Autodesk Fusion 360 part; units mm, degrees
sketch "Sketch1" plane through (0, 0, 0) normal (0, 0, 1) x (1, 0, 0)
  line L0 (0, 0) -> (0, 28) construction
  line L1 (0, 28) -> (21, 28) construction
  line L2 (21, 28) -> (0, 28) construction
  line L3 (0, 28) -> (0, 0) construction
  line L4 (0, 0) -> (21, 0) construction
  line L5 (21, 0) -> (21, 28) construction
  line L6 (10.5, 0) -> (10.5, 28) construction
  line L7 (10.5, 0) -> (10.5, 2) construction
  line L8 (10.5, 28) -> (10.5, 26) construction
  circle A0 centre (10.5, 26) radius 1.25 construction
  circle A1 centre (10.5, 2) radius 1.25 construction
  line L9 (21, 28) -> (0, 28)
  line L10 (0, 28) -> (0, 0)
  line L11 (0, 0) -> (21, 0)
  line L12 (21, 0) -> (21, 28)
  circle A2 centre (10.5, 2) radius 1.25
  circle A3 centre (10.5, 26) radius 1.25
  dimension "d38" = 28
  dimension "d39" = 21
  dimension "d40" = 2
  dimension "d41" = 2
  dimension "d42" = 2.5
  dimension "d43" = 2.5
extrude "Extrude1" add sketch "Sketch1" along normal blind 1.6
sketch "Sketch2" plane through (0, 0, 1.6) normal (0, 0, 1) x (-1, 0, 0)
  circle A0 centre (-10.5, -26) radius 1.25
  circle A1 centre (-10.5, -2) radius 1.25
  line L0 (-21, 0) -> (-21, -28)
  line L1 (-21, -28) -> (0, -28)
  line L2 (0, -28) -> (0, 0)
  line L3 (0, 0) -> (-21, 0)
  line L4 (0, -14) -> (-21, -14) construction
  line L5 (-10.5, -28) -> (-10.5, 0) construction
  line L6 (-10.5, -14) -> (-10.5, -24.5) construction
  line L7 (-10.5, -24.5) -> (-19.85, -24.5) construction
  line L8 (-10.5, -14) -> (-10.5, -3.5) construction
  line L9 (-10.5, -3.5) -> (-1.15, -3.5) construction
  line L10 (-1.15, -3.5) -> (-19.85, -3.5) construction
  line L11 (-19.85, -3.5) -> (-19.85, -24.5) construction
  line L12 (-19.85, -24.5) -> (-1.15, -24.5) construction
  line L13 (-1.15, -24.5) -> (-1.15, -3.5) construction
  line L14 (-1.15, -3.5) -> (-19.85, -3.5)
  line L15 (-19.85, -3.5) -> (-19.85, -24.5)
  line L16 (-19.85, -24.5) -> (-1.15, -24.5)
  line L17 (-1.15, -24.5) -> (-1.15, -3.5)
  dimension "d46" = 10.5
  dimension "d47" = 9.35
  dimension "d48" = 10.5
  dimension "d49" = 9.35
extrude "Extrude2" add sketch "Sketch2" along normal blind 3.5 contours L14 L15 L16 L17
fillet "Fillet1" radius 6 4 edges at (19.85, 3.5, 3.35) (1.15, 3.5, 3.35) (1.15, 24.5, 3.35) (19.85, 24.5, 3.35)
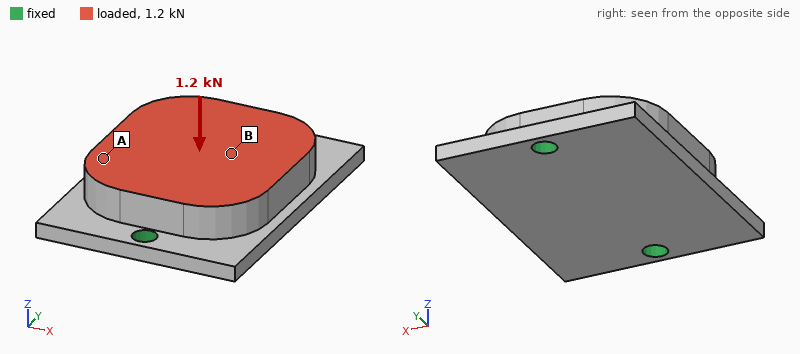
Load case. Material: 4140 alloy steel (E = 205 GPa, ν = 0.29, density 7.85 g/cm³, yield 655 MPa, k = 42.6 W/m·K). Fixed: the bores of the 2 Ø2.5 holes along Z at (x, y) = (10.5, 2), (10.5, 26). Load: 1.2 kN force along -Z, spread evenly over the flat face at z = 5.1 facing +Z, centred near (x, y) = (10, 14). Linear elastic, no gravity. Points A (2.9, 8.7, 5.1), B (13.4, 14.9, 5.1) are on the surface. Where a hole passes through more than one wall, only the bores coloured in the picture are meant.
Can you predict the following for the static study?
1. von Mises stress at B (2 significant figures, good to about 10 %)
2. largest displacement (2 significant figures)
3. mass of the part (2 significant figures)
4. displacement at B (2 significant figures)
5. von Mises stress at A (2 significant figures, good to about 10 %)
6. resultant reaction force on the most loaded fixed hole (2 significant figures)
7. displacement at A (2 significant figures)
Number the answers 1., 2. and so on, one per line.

1. 39 MPa
2. 6.6 µm
3. 17 g
4. 5.2 µm
5. 22 MPa
6. 780 N
7. 5.3 µm
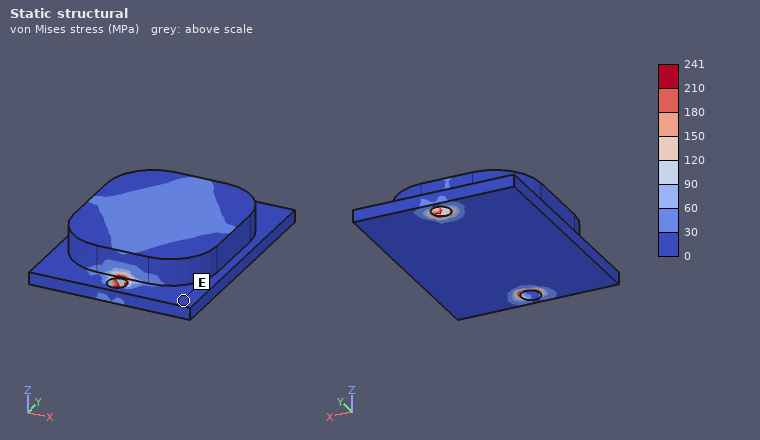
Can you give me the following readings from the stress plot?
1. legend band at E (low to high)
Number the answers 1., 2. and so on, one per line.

1. 0 to 30 MPa
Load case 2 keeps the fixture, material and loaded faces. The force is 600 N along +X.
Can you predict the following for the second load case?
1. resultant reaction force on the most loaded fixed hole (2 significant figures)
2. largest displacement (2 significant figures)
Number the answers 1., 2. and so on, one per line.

1. 300 N
2. 17 µm
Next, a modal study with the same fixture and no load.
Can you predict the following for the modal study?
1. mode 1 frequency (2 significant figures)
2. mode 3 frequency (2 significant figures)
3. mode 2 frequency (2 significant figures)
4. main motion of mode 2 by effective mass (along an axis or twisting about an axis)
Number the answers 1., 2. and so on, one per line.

1. 8300 Hz
2. 32 kHz
3. 20 kHz
4. along Z
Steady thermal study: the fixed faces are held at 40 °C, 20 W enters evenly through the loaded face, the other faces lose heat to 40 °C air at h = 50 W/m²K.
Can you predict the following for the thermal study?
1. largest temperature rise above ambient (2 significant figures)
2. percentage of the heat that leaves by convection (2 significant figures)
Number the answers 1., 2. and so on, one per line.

1. 49 K
2. 11 %
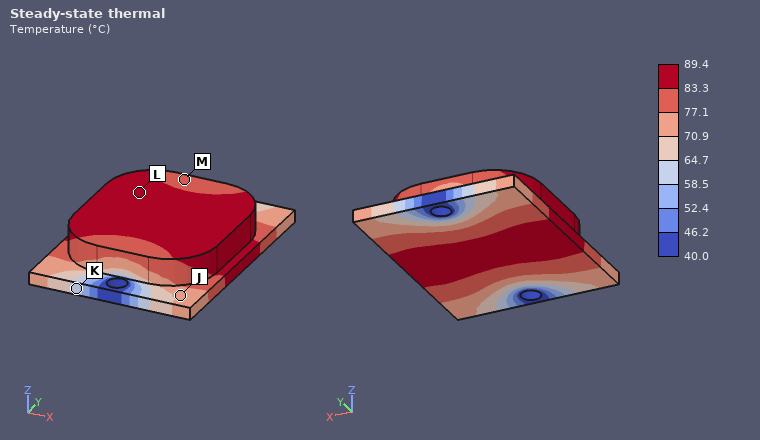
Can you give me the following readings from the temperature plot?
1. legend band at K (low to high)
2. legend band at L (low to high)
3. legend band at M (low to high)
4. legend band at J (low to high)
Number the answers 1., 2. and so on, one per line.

1. 58.5 to 64.7 °C
2. 83.3 to 89.4 °C
3. 77.1 to 83.3 °C
4. 70.9 to 77.1 °C
